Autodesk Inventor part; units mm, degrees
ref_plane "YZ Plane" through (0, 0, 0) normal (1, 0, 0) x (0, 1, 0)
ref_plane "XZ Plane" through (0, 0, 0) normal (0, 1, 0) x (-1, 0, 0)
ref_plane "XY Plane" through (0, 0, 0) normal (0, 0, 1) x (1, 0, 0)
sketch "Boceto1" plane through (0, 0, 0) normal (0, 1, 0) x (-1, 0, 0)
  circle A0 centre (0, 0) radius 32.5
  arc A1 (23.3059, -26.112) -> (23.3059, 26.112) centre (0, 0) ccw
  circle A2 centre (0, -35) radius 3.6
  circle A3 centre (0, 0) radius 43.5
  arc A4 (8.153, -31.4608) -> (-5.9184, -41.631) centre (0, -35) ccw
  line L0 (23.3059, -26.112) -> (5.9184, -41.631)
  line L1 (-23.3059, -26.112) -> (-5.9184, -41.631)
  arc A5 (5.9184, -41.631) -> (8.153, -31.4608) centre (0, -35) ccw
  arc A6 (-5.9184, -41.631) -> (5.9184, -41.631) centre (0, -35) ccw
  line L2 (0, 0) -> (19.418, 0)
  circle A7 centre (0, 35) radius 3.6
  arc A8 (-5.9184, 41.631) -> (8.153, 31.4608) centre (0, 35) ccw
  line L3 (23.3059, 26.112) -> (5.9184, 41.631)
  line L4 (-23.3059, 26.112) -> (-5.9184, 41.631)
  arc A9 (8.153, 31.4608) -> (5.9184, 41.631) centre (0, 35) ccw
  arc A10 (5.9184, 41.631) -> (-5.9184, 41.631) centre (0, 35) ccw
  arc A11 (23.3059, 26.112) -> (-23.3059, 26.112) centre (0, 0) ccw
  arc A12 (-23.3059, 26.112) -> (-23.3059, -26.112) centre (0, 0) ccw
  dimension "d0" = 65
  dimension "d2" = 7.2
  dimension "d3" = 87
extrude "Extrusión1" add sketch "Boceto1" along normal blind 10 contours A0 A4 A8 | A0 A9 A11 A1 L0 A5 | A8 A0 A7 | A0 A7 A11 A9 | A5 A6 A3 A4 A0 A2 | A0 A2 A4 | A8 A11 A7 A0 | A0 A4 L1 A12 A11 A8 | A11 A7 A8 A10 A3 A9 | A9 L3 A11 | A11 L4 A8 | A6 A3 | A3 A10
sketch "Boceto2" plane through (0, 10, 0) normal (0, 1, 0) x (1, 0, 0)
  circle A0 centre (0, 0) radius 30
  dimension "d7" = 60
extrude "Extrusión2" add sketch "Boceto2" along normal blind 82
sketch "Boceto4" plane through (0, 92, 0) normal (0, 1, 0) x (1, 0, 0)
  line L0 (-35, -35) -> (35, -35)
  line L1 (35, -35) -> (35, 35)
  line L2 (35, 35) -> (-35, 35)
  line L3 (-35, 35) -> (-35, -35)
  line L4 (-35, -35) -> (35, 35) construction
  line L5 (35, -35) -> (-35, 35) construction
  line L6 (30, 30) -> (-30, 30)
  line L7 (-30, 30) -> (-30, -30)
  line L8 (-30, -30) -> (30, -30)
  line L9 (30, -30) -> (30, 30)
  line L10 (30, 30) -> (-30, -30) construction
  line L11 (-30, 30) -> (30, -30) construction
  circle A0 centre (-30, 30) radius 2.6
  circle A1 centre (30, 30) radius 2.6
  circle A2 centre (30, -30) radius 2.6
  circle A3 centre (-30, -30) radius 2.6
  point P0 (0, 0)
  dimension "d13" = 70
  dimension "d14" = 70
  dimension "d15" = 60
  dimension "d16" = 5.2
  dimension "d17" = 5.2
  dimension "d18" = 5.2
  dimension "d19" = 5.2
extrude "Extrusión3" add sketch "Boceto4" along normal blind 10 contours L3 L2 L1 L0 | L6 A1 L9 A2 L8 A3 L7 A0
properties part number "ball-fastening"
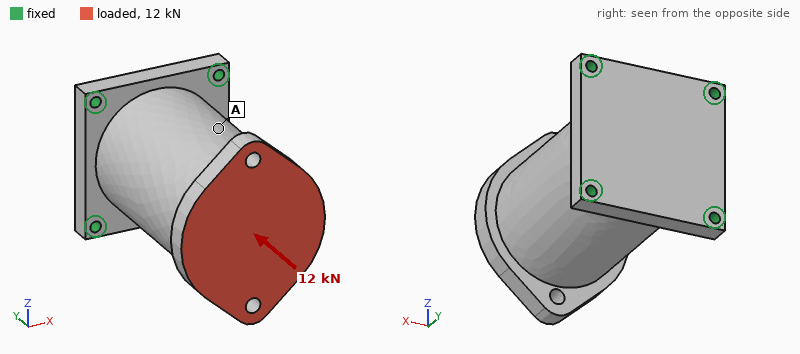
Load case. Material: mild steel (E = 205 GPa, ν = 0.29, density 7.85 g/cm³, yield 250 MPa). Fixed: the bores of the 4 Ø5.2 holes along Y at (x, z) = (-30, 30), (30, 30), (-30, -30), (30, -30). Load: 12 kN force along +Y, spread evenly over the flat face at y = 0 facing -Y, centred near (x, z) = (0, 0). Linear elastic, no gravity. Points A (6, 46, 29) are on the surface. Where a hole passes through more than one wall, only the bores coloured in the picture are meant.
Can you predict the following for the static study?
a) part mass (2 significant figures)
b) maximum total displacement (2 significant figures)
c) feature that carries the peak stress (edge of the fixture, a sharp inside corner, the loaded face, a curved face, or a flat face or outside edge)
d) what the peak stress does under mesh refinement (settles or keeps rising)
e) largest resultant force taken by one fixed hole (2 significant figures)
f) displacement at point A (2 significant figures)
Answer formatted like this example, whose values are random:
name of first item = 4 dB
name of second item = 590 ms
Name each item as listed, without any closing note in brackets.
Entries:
part mass = 2.5 kg
maximum total displacement = 11 µm
feature that carries the peak stress = edge of the fixture
what the peak stress does under mesh refinement = keeps rising
largest resultant force taken by one fixed hole = 3.1 kN
displacement at point A = 7.8 µm
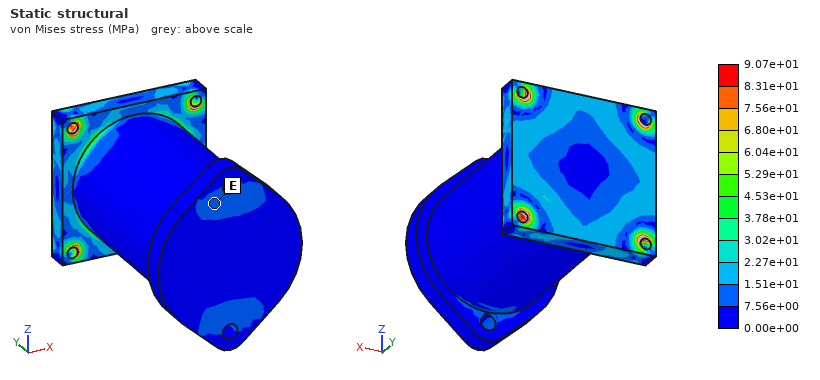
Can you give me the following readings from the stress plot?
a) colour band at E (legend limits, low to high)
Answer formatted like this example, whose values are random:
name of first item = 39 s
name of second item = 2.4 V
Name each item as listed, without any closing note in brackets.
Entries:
colour band at E = 7.56e+00 to 1.51e+01 MPa
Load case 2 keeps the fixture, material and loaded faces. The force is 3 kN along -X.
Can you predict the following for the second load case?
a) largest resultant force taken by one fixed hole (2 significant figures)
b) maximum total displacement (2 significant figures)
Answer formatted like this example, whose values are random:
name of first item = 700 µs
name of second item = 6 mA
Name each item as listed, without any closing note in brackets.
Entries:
largest resultant force taken by one fixed hole = 2.9 kN
maximum total displacement = 33 µm
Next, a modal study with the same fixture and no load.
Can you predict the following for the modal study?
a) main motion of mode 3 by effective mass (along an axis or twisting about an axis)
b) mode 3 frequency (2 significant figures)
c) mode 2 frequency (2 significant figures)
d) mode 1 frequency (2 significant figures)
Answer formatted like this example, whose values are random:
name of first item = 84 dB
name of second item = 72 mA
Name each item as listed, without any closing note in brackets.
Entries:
main motion of mode 3 by effective mass = along Y
mode 3 frequency = 4100 Hz
mode 2 frequency = 1700 Hz
mode 1 frequency = 1700 Hz
